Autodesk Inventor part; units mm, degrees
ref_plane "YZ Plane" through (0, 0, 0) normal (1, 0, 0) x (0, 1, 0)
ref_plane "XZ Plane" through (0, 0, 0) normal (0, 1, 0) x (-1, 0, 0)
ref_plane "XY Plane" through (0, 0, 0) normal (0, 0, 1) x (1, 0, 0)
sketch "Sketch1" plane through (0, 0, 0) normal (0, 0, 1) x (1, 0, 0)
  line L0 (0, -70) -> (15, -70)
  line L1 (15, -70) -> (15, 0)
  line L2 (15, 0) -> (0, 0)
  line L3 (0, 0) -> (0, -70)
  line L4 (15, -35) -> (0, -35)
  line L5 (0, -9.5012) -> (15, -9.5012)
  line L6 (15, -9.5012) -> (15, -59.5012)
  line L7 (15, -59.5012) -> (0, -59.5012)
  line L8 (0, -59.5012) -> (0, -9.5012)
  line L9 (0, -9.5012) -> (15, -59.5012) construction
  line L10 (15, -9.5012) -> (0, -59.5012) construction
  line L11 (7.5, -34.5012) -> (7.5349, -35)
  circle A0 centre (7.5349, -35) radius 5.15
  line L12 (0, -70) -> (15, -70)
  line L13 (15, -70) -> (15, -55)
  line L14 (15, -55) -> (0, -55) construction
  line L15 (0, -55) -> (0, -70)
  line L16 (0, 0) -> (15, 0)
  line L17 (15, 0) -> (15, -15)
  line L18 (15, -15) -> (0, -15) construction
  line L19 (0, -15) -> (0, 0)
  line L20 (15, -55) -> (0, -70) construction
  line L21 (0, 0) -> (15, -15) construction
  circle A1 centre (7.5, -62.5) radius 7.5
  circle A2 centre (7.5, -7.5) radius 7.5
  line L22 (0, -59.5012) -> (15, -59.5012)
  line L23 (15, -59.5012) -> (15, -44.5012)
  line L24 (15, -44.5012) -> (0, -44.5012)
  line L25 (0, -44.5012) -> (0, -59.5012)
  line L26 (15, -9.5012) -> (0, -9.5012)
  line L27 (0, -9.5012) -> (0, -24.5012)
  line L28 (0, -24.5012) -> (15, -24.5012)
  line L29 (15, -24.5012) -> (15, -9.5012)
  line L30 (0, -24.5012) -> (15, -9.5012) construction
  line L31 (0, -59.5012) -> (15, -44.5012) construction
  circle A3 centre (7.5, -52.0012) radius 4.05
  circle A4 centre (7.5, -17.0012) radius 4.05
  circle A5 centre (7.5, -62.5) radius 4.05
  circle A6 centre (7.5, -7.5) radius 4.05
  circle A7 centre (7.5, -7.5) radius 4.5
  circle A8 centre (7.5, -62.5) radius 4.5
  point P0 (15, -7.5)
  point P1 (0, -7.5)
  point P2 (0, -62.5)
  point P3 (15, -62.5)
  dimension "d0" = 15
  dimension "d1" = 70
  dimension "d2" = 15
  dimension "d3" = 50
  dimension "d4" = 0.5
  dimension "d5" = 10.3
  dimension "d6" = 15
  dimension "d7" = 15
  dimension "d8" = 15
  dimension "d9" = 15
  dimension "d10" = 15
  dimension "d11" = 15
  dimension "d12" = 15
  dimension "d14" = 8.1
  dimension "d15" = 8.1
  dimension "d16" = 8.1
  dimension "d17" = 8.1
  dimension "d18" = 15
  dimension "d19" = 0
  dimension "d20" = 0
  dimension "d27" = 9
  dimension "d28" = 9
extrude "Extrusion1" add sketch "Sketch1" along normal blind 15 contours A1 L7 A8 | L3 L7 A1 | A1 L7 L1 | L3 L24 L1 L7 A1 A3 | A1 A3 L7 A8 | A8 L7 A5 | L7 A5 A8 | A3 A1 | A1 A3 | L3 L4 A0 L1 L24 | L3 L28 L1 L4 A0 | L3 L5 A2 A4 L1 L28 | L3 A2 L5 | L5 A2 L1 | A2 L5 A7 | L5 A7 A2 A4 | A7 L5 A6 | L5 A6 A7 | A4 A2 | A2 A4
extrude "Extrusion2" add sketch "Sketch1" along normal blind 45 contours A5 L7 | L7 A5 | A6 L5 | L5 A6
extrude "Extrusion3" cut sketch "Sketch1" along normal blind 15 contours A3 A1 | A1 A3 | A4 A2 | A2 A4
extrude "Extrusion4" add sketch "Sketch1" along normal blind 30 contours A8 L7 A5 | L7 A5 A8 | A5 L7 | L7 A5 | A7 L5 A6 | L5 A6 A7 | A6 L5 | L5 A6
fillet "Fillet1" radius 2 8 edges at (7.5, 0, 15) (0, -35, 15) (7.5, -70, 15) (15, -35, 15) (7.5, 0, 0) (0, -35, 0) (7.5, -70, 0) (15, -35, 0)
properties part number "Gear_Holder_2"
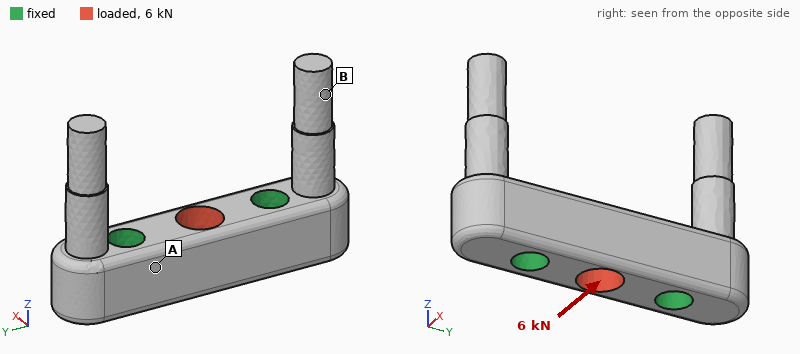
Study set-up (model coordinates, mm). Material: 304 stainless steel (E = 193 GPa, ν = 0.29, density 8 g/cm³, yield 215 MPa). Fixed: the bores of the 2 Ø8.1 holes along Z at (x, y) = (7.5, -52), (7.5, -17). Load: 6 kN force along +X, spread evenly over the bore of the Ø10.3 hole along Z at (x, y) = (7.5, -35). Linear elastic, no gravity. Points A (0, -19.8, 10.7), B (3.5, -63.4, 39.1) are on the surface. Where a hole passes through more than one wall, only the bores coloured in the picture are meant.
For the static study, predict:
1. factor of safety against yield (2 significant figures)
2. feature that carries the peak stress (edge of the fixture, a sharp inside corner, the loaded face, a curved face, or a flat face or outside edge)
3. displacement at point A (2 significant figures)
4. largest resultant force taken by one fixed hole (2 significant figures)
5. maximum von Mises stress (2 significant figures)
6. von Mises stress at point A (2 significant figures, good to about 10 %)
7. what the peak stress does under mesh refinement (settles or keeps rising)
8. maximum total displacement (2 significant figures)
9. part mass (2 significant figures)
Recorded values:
2.9
a curved face
0.83 µm
3.1 kN
74 MPa
25 MPa
settles
5.2 µm
120 g
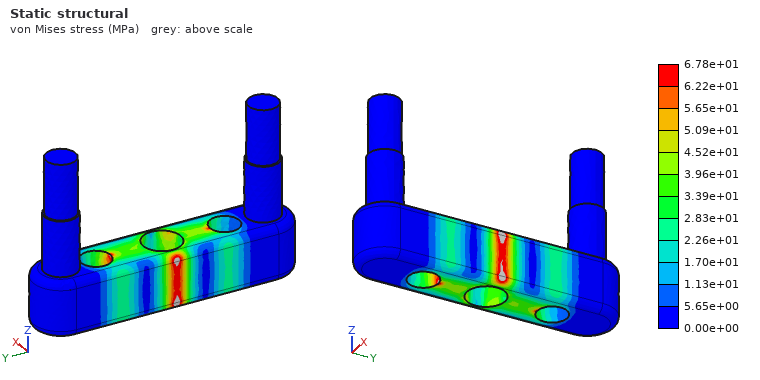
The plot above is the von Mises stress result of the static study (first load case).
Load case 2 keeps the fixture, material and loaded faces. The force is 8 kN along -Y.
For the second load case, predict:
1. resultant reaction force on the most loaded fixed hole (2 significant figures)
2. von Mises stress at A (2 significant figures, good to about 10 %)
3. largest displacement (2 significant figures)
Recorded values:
4.1 kN
9.7 MPa
1.6 µm
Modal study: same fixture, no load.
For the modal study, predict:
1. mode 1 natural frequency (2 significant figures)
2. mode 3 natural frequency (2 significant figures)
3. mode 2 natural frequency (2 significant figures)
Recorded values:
5900 Hz
6000 Hz
6000 Hz
